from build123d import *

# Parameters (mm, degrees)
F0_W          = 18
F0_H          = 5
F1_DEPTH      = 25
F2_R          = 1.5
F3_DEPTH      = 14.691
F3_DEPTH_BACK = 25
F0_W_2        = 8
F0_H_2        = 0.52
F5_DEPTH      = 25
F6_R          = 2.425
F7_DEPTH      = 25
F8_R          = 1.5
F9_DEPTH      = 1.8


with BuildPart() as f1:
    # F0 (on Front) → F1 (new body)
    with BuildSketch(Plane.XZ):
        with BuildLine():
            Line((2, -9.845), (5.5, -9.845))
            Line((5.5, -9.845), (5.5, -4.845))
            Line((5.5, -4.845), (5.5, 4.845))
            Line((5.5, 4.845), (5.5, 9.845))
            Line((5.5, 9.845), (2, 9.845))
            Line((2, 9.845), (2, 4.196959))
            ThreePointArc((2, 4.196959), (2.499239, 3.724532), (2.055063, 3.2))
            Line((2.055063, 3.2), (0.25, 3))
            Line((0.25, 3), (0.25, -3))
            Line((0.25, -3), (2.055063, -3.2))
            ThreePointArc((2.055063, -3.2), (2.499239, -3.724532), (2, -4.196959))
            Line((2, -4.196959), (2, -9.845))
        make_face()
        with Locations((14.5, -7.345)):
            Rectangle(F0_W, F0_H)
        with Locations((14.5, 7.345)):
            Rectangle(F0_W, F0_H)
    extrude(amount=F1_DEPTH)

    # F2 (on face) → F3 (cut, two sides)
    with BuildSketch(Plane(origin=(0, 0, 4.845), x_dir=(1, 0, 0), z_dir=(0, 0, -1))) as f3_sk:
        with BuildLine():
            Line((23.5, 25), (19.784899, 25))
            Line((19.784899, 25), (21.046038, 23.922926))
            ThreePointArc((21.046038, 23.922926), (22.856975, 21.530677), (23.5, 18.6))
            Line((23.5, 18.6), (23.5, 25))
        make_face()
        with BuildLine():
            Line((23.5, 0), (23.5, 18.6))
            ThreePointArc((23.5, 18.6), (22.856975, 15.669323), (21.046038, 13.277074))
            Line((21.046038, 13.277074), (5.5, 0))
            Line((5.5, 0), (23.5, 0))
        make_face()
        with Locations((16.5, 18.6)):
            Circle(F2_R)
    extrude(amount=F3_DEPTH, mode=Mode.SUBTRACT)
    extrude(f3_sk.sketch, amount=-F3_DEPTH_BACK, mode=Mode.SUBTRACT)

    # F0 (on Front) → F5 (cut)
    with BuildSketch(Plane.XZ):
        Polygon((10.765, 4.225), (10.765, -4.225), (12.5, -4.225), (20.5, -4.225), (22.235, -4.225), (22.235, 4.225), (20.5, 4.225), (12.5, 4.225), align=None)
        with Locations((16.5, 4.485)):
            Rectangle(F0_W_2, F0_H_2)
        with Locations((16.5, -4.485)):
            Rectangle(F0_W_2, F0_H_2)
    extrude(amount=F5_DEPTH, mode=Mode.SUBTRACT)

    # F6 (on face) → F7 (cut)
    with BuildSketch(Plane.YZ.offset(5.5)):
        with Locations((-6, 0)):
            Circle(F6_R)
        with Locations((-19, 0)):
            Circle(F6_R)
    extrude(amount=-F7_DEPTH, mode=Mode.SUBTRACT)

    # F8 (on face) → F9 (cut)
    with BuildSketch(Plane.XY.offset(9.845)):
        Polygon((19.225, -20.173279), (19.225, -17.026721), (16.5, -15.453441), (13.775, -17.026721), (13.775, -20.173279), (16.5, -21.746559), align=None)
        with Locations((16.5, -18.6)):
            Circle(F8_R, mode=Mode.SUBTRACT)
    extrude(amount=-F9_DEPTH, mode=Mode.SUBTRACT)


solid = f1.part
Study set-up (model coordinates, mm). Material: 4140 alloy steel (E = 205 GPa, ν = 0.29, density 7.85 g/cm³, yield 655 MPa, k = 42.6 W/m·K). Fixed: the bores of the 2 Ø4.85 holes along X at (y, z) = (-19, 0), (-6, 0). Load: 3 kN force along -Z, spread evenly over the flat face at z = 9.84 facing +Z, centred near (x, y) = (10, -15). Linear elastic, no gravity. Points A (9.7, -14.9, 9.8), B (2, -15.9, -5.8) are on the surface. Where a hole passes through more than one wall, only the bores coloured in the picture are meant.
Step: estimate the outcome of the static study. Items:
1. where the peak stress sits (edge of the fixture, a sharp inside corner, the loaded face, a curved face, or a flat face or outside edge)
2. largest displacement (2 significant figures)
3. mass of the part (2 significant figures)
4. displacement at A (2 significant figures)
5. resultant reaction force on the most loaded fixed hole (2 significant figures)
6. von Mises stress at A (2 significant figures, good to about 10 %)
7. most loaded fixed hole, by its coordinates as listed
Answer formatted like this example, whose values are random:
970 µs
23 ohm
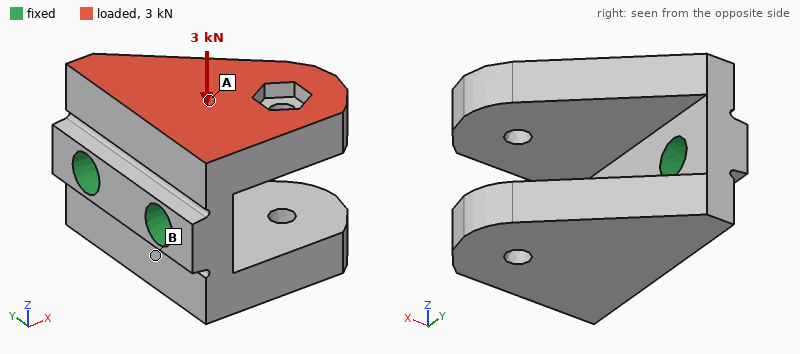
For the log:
a curved face
0.16 mm
37 g
0.057 mm
1.9 kN
98 MPa
(-19, 0)
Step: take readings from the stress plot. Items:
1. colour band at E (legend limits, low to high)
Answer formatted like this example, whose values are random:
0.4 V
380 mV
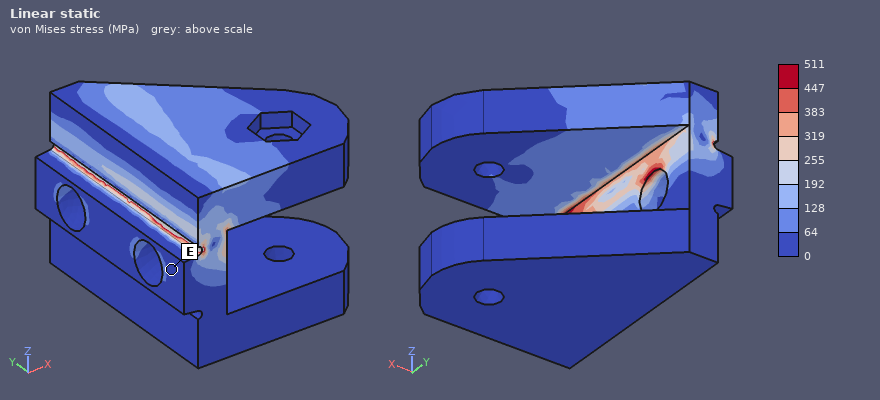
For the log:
0 to 64 MPa
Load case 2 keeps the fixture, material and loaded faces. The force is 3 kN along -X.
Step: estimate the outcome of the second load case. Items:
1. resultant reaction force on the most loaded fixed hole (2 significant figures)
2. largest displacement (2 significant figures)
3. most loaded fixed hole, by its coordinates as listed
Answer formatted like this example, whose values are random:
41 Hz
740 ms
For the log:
1.9 kN
0.13 mm
(-19, 0)
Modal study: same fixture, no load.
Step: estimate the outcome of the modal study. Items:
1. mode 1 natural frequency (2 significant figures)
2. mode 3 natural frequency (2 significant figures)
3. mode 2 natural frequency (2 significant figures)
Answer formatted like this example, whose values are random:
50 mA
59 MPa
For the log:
6800 Hz
17 kHz
7000 Hz
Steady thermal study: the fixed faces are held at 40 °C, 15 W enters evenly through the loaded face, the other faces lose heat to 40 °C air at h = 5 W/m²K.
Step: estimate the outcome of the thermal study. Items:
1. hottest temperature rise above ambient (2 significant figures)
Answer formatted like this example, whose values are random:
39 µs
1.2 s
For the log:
48 K
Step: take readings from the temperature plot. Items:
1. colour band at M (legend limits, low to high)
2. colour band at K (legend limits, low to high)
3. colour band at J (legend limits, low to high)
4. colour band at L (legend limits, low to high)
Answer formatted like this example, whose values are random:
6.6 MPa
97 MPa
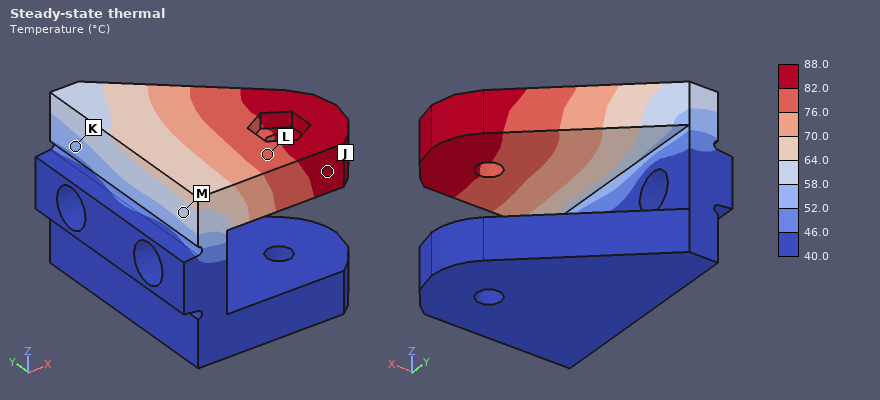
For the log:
58.0 to 64.0 °C
52.0 to 58.0 °C
82.0 to 88.0 °C
76.0 to 82.0 °C
